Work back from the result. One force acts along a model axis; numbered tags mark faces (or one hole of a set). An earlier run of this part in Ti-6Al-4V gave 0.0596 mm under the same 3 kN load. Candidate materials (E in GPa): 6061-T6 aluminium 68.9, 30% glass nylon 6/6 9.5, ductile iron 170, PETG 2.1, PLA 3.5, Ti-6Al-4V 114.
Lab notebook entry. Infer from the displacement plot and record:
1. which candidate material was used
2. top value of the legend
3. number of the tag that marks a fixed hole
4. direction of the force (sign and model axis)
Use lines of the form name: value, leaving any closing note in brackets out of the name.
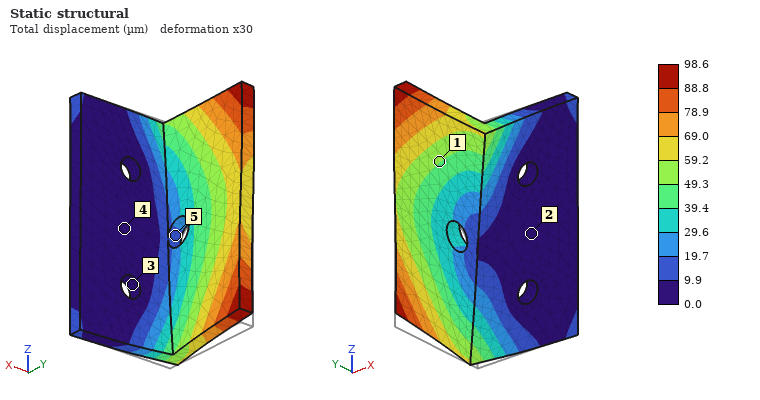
which candidate material was used: 6061-T6 aluminium
top value of the legend: 98.6 µm
number of the tag that marks a fixed hole: 3
direction of the force: +Z
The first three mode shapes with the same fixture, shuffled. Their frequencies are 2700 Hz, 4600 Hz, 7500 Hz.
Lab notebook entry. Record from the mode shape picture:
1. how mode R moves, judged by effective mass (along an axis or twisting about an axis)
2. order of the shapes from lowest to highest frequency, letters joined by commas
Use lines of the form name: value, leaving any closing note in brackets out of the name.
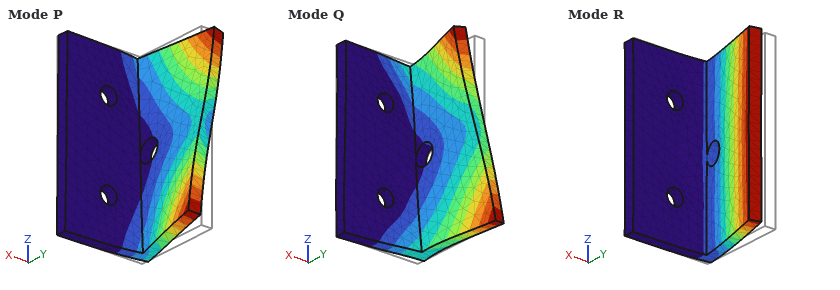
how mode R moves, judged by effective mass: along X
order of the shapes from lowest to highest frequency, letters joined by commas: R, P, Q
